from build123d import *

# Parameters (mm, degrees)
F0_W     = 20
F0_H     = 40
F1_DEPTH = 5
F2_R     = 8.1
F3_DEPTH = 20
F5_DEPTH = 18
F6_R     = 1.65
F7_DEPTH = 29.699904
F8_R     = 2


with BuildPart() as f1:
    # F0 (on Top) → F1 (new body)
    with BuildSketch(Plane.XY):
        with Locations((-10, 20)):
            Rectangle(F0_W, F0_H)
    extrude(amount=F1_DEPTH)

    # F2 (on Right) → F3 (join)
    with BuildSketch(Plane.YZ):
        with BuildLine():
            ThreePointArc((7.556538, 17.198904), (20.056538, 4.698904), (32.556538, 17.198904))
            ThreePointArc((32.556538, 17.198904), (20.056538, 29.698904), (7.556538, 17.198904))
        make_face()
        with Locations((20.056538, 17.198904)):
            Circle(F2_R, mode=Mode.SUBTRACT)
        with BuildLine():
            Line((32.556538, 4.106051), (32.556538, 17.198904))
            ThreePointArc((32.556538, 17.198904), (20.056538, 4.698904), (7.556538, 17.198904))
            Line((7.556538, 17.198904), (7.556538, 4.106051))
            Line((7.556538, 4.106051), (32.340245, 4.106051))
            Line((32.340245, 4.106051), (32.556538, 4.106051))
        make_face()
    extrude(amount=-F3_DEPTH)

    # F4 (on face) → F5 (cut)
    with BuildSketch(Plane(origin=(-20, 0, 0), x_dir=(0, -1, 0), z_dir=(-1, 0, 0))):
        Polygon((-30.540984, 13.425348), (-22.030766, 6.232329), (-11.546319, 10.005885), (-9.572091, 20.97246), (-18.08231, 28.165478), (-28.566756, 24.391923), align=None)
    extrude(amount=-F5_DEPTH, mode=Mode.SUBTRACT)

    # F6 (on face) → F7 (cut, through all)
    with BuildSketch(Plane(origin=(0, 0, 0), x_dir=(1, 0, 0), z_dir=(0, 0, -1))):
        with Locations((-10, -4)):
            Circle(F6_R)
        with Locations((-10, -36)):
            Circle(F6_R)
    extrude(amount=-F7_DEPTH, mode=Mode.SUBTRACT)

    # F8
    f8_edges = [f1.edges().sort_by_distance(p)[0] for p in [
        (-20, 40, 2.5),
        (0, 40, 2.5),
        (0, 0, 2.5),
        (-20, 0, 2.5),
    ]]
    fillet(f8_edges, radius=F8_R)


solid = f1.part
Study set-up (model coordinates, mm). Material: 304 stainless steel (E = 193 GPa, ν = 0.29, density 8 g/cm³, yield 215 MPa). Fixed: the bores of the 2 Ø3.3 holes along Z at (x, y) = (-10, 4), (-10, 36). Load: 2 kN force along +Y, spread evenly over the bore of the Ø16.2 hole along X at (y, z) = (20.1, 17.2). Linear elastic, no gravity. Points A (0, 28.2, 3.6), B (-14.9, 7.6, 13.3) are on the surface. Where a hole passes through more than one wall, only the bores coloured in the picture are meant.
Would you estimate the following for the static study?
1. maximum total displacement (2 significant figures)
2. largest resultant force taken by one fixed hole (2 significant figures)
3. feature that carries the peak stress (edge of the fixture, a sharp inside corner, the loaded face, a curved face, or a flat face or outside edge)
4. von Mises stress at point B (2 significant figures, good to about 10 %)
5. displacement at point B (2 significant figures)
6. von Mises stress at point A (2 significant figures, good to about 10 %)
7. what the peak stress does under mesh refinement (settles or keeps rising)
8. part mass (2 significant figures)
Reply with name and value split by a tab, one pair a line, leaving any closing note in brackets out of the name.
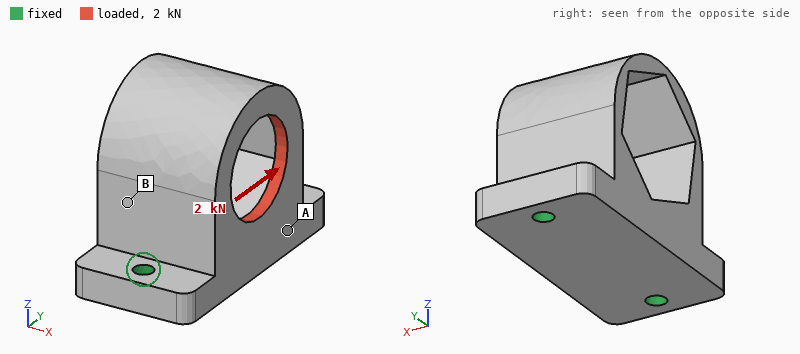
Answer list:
maximum total displacement	29 µm
largest resultant force taken by one fixed hole	1.5 kN
feature that carries the peak stress	a sharp inside corner
von Mises stress at point B	57 MPa
displacement at point B	6.3 µm
von Mises stress at point A	19 MPa
what the peak stress does under mesh refinement	keeps rising
part mass	69 g
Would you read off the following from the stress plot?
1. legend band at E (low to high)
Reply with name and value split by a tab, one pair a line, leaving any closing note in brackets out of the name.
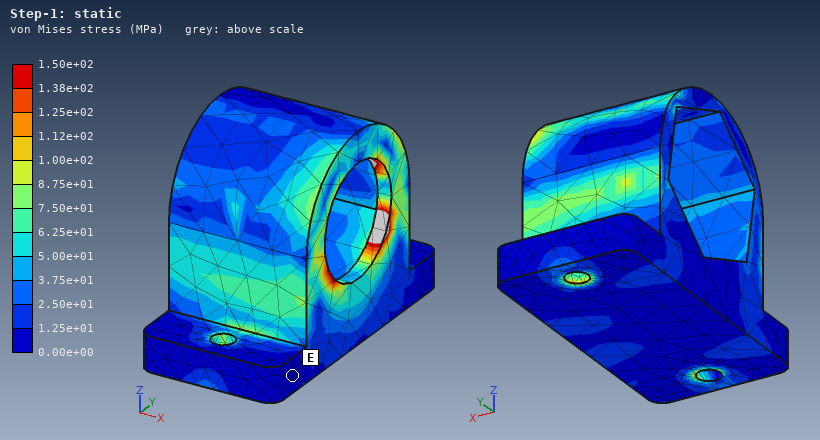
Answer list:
legend band at E	0.00e+00 to 1.25e+01 MPa
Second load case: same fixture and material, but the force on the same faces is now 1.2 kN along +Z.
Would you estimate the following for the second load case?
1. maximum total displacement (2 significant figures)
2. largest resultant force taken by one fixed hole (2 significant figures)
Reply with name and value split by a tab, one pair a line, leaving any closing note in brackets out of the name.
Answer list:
maximum total displacement	23 µm
largest resultant force taken by one fixed hole	640 N
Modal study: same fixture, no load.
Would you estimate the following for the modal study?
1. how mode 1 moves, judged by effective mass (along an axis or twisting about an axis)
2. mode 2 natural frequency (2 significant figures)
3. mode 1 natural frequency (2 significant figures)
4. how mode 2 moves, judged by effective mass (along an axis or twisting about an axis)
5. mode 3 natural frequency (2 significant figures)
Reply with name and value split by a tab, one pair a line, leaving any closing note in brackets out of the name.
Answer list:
how mode 1 moves, judged by effective mass	along X
mode 2 natural frequency	8500 Hz
mode 1 natural frequency	6100 Hz
how mode 2 moves, judged by effective mass	along Y
mode 3 natural frequency	16 kHz
